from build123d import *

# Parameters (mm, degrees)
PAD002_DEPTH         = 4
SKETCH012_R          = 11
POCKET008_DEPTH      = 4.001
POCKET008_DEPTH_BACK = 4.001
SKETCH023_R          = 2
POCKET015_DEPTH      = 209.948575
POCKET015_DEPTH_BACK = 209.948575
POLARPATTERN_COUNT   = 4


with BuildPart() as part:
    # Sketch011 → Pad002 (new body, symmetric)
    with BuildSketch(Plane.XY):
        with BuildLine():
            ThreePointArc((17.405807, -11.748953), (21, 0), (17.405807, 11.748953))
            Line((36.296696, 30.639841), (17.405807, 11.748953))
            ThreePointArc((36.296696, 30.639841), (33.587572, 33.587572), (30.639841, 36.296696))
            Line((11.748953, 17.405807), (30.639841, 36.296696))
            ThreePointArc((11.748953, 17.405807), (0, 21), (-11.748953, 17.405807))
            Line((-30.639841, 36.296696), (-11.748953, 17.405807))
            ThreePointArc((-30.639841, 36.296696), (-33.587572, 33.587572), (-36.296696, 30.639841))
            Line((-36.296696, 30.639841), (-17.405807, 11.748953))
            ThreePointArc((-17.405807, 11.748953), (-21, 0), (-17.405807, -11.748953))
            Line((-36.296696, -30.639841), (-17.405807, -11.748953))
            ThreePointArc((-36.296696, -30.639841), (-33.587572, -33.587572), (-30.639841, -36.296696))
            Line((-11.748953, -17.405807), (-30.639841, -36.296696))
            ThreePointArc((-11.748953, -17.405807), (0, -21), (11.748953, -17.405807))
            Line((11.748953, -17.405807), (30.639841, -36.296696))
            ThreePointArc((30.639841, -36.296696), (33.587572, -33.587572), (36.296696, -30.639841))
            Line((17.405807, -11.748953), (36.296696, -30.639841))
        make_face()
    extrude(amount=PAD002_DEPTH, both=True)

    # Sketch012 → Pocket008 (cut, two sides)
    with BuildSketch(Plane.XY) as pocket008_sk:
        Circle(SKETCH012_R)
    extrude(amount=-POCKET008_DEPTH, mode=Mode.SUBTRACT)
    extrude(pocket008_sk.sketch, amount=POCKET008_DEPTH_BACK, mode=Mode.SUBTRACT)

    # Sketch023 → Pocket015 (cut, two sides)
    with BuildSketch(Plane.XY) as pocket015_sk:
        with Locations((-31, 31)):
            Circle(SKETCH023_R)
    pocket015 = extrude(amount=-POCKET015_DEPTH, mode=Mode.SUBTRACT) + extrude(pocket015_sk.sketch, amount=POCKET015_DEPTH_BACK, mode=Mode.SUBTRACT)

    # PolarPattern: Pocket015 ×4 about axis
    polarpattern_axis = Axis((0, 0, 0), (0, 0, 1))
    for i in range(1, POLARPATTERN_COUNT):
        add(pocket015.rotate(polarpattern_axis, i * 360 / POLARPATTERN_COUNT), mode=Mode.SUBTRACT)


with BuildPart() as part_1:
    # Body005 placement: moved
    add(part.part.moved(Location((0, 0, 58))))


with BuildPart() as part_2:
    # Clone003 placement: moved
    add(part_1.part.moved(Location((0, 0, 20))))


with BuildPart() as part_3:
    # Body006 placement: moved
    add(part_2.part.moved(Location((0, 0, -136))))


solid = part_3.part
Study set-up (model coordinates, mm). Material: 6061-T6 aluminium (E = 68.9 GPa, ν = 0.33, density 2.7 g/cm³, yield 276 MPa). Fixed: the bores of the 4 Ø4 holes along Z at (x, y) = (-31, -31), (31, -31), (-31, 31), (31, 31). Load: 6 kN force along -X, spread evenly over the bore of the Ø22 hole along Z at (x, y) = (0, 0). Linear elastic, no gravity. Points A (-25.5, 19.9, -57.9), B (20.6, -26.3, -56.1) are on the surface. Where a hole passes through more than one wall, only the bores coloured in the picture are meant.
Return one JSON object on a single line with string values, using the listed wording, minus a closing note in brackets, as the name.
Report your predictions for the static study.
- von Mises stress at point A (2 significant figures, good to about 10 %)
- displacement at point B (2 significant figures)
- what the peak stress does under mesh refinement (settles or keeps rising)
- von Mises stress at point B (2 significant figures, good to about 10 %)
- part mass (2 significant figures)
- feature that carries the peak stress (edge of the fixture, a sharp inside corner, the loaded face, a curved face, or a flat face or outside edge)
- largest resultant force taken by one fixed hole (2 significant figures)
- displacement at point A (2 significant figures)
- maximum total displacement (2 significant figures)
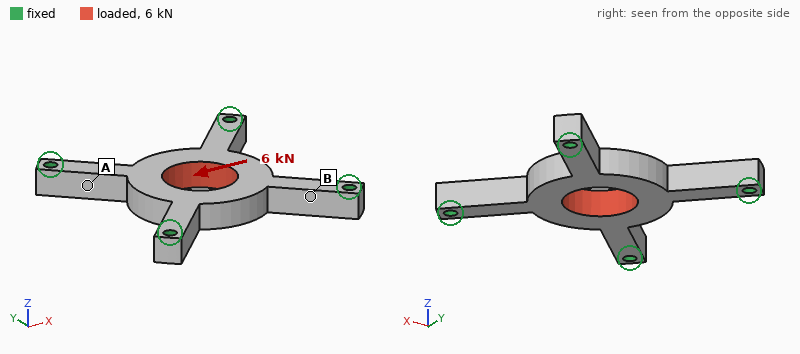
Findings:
{"von Mises stress at point A": "35 MPa", "displacement at point B": "4.8 µm", "what the peak stress does under mesh refinement": "keeps rising", "von Mises stress at point B": "25 MPa", "part mass": "39 g", "feature that carries the peak stress": "edge of the fixture", "largest resultant force taken by one fixed hole": "2.0 kN", "displacement at point A": "9.9 µm", "maximum total displacement": "25 µm"}
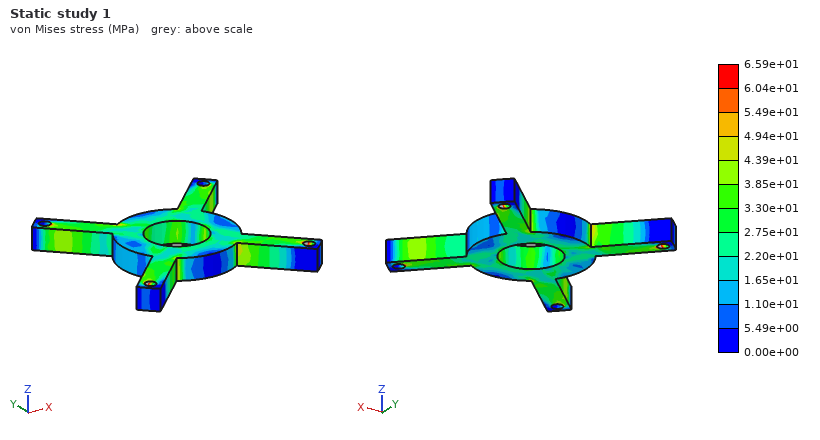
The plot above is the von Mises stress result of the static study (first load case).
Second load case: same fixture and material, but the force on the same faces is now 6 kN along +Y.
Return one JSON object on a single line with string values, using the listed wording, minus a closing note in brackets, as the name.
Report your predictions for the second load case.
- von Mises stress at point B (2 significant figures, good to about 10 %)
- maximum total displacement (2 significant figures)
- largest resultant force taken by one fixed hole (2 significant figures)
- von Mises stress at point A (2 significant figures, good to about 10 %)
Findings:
{"von Mises stress at point B": "37 MPa", "maximum total displacement": "25 µm", "largest resultant force taken by one fixed hole": "2.0 kN", "von Mises stress at point A": "26 MPa"}
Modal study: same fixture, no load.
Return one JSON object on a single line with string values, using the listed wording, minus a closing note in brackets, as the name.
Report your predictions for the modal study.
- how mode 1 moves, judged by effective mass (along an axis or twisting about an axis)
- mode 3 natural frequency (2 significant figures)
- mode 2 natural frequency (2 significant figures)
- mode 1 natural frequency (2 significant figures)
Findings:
{"how mode 1 moves, judged by effective mass": "along Z", "mode 3 natural frequency": "10 kHz", "mode 2 natural frequency": "10 kHz", "mode 1 natural frequency": "5700 Hz"}
